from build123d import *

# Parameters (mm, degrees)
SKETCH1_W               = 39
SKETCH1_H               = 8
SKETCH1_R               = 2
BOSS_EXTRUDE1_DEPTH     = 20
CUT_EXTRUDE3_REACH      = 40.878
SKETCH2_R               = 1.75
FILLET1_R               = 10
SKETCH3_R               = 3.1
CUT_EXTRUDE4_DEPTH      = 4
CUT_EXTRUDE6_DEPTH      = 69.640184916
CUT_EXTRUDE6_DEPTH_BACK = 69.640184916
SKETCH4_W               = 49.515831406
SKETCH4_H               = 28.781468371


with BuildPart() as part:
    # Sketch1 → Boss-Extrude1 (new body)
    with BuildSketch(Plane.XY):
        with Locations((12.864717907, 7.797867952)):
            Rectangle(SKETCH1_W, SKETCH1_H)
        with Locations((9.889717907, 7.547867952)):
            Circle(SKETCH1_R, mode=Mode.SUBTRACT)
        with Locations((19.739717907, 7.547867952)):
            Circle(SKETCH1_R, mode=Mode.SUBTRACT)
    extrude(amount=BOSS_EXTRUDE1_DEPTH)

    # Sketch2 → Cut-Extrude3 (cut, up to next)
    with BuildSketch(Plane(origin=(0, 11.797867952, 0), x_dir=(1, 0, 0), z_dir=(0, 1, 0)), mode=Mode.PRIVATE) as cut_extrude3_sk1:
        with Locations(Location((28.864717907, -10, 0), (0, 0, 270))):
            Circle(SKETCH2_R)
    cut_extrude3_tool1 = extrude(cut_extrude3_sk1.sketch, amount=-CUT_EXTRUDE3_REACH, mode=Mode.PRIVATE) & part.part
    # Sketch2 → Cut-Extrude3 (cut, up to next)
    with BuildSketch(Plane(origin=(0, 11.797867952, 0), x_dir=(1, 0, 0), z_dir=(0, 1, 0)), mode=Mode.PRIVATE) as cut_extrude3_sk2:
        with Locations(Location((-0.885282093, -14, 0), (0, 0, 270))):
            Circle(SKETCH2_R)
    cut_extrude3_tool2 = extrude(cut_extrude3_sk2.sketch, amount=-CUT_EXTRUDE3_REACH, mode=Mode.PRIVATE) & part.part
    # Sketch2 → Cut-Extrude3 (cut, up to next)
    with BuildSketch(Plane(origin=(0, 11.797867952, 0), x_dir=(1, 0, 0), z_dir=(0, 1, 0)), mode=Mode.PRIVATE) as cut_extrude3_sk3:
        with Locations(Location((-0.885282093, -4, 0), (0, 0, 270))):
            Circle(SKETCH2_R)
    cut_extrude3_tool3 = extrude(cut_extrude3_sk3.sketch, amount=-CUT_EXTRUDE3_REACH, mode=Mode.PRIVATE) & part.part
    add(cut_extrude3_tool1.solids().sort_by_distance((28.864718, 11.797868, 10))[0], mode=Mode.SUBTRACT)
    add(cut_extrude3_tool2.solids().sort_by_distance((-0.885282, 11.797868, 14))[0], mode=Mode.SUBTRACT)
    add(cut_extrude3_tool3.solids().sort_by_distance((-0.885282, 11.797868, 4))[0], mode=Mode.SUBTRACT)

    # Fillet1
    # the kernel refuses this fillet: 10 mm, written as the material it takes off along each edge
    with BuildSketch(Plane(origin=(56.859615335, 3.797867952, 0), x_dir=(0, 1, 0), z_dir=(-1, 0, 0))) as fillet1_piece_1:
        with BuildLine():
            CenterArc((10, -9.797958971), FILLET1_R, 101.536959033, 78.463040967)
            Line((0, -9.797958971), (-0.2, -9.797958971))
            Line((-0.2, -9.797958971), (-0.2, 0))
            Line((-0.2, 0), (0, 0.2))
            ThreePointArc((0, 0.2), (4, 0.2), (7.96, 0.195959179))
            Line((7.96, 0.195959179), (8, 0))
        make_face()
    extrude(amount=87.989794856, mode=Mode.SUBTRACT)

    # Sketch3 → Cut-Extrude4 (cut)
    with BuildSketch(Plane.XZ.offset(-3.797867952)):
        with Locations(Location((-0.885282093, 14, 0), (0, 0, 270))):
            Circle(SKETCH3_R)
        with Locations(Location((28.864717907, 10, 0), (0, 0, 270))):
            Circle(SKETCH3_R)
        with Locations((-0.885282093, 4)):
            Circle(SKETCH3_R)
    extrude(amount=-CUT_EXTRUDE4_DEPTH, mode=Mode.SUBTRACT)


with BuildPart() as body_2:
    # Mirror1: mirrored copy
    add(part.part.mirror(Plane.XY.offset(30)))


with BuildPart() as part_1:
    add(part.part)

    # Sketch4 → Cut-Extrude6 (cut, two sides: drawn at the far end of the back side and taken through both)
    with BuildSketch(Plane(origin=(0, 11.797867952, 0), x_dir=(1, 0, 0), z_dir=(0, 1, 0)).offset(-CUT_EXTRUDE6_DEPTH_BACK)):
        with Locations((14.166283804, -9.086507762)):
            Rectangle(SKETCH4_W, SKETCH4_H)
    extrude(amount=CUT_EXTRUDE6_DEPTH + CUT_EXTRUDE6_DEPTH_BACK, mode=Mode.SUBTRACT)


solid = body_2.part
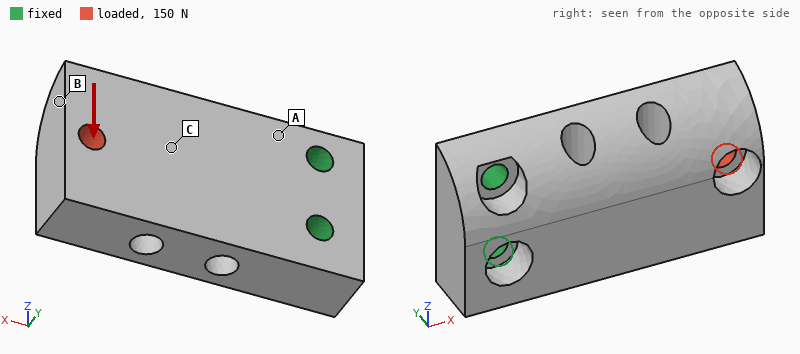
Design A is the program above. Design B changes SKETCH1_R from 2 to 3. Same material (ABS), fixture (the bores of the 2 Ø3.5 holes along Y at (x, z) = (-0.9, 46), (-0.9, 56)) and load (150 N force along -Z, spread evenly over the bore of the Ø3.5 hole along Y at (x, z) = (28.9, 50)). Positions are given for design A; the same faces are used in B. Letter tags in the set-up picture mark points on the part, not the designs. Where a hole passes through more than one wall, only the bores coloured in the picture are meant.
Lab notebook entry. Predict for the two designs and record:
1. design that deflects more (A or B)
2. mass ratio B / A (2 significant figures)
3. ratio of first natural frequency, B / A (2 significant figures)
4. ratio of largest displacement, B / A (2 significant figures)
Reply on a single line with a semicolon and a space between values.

B; 0.88; 0.93; 1.4
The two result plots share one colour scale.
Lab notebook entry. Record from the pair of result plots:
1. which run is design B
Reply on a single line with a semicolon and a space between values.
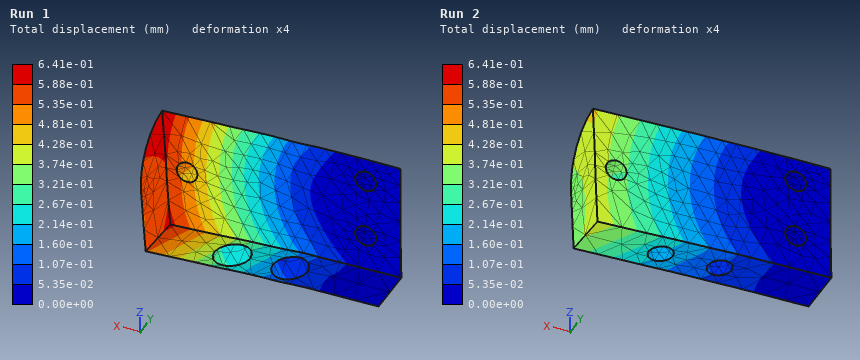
Run 1
